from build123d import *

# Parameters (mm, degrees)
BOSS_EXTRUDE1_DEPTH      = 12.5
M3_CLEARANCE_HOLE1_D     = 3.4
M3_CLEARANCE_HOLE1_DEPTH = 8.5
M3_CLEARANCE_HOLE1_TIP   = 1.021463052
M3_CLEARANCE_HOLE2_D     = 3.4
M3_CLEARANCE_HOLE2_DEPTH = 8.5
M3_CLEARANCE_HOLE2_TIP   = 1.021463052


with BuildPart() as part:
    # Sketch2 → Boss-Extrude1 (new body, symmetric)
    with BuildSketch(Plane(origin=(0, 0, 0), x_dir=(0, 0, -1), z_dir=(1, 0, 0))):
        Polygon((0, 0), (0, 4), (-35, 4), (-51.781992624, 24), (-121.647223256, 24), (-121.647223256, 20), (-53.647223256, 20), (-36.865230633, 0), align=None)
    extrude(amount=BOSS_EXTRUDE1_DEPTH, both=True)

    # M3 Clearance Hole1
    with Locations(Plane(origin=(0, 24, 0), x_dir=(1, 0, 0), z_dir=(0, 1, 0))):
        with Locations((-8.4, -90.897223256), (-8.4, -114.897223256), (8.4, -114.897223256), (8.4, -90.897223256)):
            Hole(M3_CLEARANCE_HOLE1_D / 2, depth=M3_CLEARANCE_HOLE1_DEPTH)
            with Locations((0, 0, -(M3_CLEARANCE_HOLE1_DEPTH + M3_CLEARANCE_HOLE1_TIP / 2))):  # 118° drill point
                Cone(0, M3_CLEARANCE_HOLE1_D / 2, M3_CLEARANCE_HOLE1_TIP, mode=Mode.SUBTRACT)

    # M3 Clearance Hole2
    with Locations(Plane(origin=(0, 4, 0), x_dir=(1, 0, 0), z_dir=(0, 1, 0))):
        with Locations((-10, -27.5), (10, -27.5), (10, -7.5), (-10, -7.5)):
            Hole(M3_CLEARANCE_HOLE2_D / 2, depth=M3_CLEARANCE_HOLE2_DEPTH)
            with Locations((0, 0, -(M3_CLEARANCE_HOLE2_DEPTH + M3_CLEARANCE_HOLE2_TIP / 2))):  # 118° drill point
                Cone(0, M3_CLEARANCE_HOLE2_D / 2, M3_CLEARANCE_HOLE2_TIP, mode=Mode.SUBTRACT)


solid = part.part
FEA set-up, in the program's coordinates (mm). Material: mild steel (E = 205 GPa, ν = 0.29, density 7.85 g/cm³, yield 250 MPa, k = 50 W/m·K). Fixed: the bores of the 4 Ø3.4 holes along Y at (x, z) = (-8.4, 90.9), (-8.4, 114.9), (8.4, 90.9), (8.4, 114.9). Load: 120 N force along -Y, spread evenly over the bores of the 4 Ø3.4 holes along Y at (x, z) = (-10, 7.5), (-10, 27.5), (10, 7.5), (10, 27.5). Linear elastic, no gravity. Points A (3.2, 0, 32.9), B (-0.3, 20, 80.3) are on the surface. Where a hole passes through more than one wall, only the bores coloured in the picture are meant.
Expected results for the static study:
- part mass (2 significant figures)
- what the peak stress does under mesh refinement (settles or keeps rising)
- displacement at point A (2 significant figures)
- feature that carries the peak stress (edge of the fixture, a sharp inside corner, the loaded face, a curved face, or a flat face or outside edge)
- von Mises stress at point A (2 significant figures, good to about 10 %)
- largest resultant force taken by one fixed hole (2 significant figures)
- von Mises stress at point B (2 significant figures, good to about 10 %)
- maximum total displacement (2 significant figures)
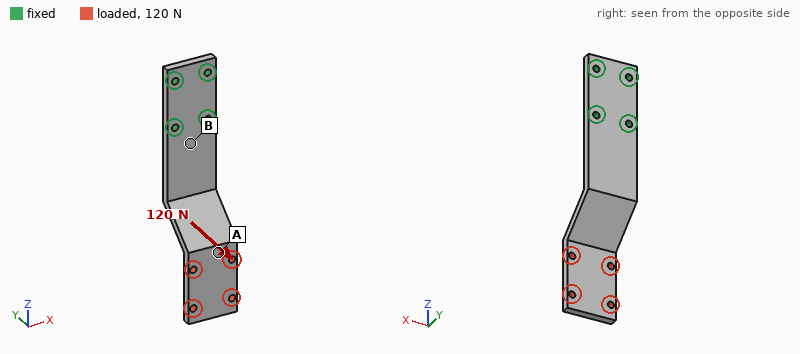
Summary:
100 g
keeps rising
0.46 mm
edge of the fixture
25 MPa
89 N
110 MPa
0.85 mm
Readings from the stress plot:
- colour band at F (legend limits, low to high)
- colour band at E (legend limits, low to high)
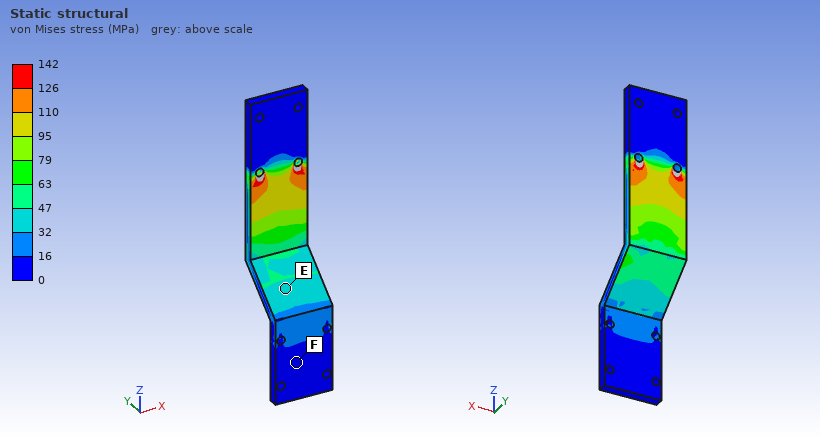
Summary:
0 to 16 MPa
32 to 47 MPa
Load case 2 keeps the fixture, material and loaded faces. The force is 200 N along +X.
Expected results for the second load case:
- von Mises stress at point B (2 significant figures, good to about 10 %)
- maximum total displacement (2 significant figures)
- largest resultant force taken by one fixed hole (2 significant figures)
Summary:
51 MPa
0.13 mm
810 N
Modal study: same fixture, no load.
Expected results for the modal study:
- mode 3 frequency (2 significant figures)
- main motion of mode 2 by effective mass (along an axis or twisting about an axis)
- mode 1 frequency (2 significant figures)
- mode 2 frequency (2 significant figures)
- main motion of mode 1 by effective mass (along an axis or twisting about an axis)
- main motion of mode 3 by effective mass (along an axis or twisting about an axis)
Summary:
2100 Hz
along X
370 Hz
1200 Hz
along Y
along Y
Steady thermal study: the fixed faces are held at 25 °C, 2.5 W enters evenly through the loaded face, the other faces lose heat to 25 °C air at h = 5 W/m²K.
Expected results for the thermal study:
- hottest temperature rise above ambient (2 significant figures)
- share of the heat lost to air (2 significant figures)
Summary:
35 K
23 %
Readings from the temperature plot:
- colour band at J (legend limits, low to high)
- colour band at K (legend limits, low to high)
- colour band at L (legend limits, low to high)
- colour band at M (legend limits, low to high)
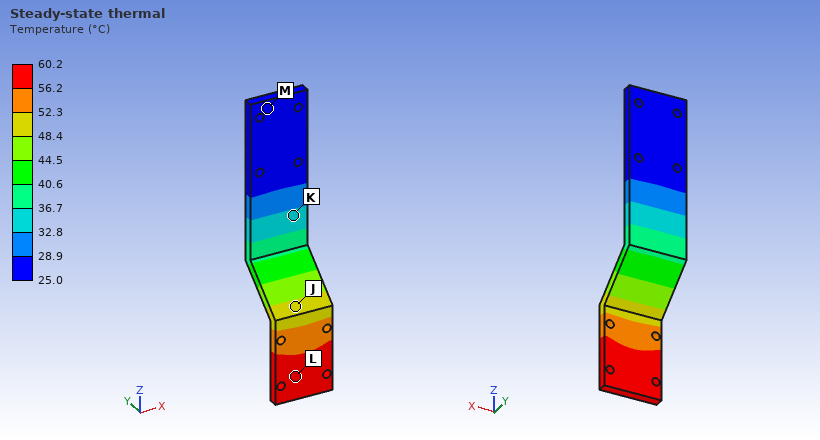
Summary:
48.4 to 52.3 °C
32.8 to 36.7 °C
56.2 to 60.2 °C
25.0 to 28.9 °C
